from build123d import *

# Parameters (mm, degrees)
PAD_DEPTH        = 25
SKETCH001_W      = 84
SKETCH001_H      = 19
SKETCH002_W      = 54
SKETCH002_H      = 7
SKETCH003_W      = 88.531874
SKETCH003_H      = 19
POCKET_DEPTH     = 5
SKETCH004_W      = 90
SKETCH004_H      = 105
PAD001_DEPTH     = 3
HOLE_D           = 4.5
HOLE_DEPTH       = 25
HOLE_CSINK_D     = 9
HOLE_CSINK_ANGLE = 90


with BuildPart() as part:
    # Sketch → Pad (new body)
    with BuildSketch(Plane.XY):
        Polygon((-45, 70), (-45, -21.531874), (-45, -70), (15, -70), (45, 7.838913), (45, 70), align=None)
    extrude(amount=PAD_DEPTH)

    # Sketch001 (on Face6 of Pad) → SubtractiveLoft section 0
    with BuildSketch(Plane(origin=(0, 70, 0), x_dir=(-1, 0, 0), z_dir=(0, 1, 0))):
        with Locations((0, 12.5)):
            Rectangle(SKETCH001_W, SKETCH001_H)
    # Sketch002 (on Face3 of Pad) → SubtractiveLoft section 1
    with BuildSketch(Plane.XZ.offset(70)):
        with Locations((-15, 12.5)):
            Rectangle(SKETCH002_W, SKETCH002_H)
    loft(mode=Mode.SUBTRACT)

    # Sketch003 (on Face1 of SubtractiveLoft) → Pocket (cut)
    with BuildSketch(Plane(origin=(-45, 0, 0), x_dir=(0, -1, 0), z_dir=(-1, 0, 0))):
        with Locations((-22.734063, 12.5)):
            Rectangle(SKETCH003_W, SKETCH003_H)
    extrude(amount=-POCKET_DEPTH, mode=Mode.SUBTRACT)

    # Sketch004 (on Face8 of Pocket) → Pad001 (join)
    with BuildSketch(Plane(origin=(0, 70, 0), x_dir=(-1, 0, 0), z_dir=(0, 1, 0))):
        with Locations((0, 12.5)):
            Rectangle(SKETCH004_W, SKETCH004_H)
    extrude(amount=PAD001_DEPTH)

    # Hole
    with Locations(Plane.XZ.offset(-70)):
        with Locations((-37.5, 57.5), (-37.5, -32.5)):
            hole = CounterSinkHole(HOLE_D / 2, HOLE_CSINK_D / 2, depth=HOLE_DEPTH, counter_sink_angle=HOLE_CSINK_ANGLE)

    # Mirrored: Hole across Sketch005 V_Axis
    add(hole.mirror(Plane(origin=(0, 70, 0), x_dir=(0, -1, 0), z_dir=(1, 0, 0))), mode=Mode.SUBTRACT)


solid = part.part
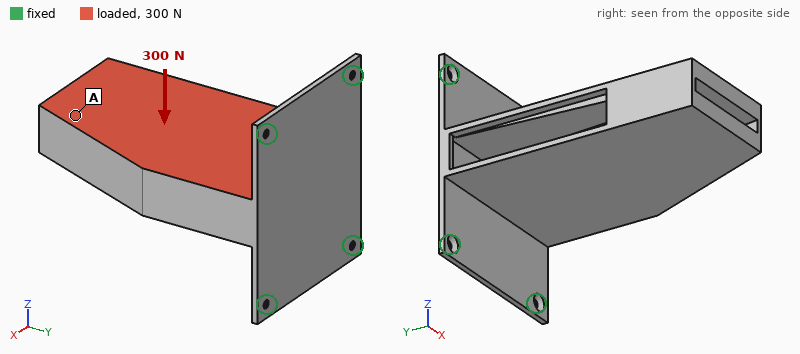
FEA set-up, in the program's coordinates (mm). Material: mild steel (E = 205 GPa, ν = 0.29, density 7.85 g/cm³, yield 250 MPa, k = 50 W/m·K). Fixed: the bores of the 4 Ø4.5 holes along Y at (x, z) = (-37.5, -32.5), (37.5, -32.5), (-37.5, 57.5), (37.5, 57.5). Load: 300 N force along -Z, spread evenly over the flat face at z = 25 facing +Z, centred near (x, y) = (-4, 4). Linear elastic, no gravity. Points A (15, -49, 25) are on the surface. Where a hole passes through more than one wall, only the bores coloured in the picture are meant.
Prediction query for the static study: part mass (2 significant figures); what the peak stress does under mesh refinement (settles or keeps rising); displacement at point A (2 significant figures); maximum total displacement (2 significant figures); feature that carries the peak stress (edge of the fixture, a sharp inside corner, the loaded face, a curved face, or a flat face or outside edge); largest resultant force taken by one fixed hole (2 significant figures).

1.4 kg
keeps rising
0.19 mm
0.23 mm
edge of the fixture
220 N
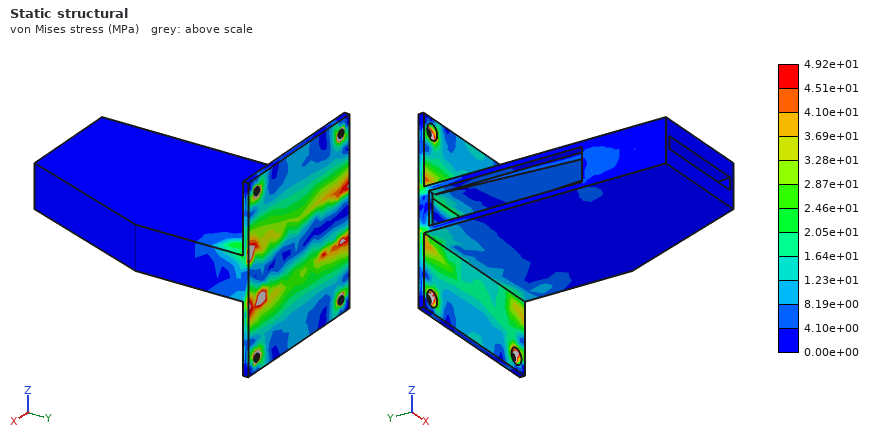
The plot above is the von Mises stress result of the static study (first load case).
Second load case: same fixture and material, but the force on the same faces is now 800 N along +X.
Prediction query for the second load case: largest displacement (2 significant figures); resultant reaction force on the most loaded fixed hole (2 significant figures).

0.52 mm
1.1 kN
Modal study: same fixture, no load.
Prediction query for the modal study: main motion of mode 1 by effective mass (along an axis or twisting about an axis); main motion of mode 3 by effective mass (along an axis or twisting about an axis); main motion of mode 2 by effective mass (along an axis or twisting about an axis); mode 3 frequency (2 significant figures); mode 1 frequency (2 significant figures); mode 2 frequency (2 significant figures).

along Z
along Y
along X
460 Hz
190 Hz
200 Hz
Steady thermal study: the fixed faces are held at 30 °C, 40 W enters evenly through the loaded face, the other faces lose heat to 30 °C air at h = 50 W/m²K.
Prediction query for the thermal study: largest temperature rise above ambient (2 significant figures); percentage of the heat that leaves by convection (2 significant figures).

28 K
91 %
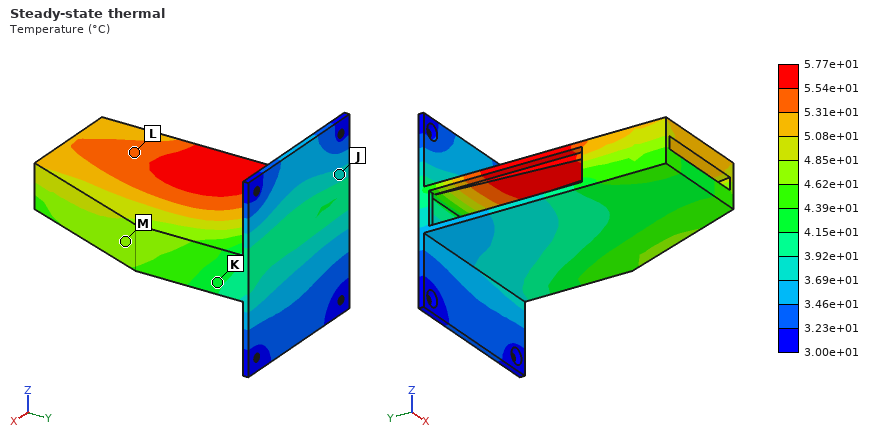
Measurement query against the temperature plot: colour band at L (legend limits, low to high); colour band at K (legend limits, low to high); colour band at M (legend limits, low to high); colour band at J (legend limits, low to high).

5.31e+01 to 5.54e+01 °C
4.15e+01 to 4.39e+01 °C
4.62e+01 to 4.85e+01 °C
3.69e+01 to 3.92e+01 °C
